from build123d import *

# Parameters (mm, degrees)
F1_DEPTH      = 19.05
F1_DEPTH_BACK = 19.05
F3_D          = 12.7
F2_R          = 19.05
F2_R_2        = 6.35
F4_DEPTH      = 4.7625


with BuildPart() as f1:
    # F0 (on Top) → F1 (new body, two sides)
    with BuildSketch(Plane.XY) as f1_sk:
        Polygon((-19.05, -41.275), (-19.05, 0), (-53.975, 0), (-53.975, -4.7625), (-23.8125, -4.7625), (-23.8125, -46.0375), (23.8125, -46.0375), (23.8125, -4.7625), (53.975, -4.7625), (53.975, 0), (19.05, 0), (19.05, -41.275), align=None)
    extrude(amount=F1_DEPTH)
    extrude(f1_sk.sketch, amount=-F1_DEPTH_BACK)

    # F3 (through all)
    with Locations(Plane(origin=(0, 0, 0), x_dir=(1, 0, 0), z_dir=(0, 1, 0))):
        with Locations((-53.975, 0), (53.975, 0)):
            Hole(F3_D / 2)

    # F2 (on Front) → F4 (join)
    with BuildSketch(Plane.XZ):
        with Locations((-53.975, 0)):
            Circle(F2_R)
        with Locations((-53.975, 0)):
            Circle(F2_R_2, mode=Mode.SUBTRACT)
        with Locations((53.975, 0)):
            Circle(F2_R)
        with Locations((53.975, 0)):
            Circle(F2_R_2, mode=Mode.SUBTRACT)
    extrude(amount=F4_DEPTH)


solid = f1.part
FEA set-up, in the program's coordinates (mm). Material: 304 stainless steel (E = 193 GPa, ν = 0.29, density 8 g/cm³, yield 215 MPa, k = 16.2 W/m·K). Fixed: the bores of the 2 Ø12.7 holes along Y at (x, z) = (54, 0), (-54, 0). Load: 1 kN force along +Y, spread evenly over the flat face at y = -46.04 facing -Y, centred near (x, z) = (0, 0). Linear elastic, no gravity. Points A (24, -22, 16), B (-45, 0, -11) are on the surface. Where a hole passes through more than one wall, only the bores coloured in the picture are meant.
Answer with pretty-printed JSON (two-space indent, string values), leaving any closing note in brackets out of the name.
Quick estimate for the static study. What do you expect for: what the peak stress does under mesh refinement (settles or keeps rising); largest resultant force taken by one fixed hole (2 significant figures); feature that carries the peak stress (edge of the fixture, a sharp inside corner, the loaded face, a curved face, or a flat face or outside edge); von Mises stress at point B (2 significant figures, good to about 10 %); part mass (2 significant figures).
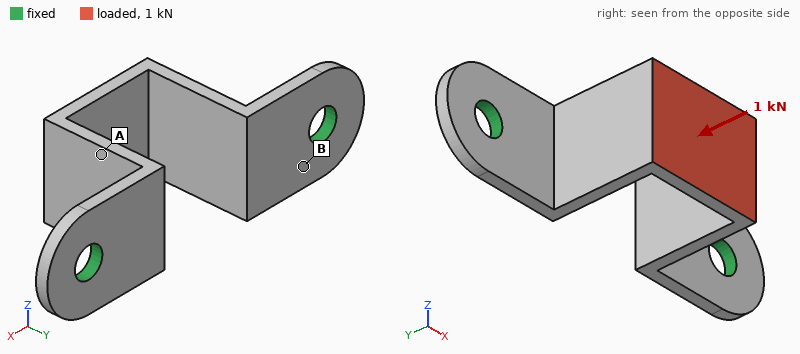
{
  "what the peak stress does under mesh refinement": "keeps rising",
  "largest resultant force taken by one fixed hole": "540 N",
  "feature that carries the peak stress": "edge of the fixture",
  "von Mises stress at point B": "31 MPa",
  "part mass": "310 g"
}
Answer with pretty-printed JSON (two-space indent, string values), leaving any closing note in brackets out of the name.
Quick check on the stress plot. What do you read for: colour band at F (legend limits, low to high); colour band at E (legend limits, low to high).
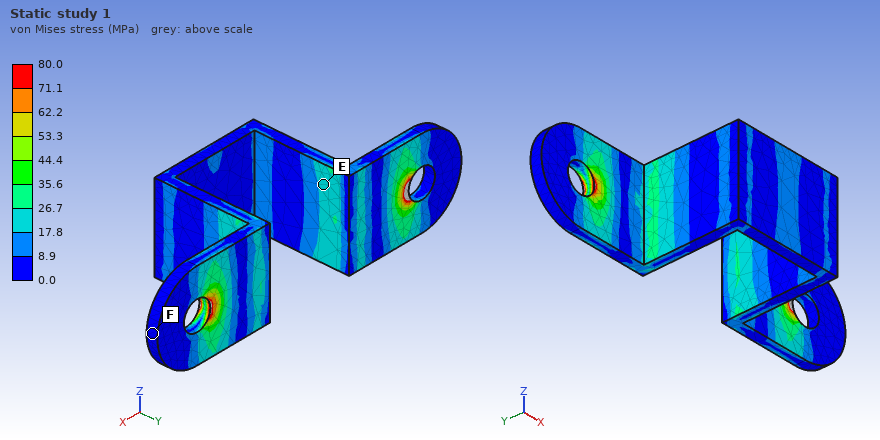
{
  "colour band at F": "0.0 to 8.9 MPa",
  "colour band at E": "17.8 to 26.7 MPa"
}
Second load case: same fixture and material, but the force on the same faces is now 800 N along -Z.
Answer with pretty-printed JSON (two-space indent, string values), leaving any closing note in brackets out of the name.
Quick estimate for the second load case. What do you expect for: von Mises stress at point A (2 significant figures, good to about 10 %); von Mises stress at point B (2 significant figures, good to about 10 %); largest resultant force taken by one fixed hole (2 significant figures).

{
  "von Mises stress at point A": "16 MPa",
  "von Mises stress at point B": "70 MPa",
  "largest resultant force taken by one fixed hole": "400 N"
}
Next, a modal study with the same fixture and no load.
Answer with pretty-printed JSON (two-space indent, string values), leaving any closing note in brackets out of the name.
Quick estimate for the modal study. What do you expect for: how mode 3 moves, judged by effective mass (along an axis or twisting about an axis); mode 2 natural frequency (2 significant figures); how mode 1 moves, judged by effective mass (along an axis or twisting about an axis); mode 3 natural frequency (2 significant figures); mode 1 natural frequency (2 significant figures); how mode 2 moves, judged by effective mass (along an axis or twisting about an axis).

{
  "how mode 3 moves, judged by effective mass": "along Y",
  "mode 2 natural frequency": "1700 Hz",
  "how mode 1 moves, judged by effective mass": "along Z",
  "mode 3 natural frequency": "2100 Hz",
  "mode 1 natural frequency": "1100 Hz",
  "how mode 2 moves, judged by effective mass": "along X"
}
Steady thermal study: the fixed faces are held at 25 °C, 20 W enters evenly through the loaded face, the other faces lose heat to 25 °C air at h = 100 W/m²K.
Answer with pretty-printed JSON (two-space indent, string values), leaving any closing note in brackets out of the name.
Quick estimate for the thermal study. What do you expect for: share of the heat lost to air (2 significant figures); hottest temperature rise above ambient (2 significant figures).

{
  "share of the heat lost to air": "98 %",
  "hottest temperature rise above ambient": "52 K"
}
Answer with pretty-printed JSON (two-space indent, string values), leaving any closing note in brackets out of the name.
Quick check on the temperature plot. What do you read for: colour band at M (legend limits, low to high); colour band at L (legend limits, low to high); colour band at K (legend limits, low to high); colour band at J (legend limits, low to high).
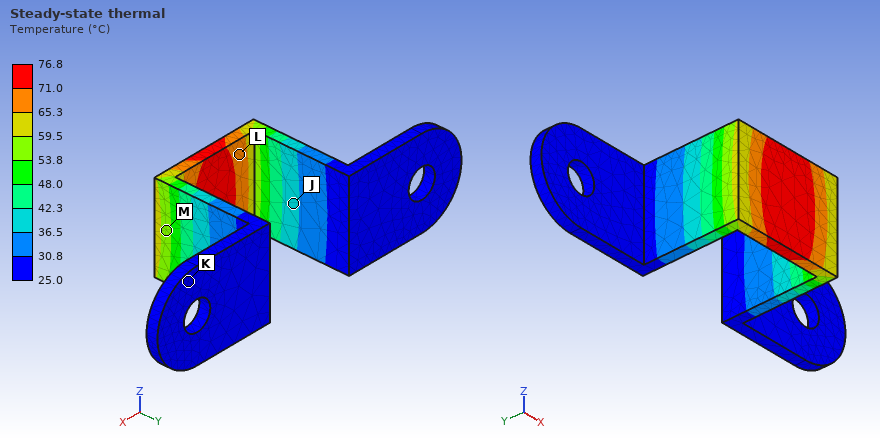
{
  "colour band at M": "53.8 to 59.5 °C",
  "colour band at L": "65.3 to 71.0 °C",
  "colour band at K": "25.0 to 30.8 °C",
  "colour band at J": "36.5 to 42.3 °C"
}
